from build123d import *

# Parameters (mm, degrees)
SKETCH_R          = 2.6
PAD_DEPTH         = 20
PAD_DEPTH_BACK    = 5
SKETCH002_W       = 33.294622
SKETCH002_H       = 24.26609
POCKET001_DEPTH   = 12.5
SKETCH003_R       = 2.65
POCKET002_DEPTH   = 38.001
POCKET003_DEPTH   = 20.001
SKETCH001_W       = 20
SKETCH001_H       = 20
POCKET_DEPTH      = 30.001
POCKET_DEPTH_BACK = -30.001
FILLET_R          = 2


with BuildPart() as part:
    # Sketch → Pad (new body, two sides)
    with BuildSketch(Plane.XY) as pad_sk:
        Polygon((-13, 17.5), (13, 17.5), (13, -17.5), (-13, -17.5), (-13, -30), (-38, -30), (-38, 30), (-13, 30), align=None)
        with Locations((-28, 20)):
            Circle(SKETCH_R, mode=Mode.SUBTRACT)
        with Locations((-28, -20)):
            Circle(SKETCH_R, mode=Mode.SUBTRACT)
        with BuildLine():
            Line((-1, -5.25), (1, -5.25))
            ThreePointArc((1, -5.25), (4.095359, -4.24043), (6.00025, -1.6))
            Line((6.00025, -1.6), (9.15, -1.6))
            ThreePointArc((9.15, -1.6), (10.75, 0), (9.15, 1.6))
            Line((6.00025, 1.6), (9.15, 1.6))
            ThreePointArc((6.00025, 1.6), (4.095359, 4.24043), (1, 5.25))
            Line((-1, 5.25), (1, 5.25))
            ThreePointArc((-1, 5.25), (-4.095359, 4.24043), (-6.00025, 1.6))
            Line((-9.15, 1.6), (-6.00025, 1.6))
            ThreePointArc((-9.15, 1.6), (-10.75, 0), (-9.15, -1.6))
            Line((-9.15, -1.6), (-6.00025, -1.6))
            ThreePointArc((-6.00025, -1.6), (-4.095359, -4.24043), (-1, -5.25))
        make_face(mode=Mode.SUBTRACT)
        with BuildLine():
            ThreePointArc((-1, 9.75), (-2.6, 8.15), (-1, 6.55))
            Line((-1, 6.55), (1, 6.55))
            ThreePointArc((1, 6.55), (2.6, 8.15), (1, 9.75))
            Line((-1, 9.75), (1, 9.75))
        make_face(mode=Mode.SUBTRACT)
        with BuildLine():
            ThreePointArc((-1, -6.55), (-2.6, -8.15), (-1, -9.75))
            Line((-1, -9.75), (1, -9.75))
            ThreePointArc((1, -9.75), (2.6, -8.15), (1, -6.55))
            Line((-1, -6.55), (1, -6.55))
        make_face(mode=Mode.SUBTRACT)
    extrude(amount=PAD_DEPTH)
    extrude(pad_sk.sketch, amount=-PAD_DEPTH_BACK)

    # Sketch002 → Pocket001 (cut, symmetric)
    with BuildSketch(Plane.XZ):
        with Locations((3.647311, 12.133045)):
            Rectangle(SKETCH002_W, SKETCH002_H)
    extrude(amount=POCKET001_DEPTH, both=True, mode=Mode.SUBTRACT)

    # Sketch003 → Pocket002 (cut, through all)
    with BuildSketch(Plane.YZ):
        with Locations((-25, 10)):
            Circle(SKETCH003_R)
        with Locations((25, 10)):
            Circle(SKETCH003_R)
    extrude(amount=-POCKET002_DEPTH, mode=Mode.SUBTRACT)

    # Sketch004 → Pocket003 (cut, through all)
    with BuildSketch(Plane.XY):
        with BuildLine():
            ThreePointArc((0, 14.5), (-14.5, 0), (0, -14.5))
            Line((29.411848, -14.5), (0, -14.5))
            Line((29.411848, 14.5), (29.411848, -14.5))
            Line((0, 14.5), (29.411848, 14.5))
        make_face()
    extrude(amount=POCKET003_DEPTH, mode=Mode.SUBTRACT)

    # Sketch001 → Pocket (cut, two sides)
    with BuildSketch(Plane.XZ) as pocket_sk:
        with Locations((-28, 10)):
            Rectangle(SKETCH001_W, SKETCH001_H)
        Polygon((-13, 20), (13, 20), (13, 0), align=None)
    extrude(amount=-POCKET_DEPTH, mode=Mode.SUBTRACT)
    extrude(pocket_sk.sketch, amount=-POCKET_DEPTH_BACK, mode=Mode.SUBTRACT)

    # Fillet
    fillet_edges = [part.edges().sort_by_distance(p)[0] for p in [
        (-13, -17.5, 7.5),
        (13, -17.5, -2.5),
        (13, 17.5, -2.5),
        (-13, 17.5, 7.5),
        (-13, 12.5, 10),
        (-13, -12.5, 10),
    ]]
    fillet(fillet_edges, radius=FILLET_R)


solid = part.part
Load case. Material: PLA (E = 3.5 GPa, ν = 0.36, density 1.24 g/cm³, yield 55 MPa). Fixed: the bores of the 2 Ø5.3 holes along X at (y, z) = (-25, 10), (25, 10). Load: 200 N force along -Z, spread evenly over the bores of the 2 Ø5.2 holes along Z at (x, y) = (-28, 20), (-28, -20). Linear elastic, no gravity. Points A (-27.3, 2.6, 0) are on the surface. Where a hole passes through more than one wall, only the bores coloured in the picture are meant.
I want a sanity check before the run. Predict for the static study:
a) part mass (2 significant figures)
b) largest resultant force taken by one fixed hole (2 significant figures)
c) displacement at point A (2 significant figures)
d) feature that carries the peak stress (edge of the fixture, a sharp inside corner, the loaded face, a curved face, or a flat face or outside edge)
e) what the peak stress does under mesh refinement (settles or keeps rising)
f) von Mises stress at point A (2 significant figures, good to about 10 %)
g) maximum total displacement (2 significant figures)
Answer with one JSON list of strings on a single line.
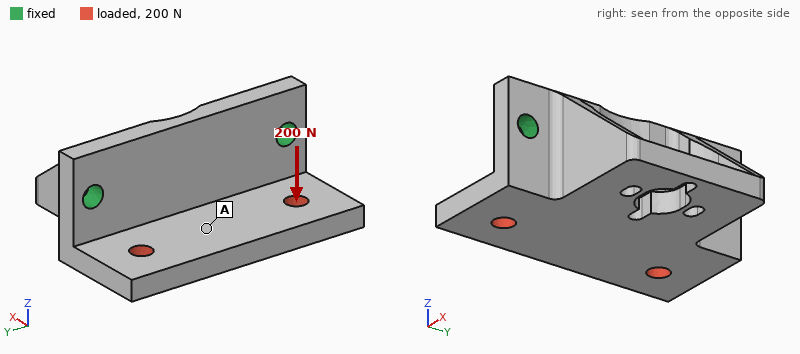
["23 g", "110 N", "0.17 mm", "edge of the fixture", "keeps rising", "2.5 MPa", "0.39 mm"]
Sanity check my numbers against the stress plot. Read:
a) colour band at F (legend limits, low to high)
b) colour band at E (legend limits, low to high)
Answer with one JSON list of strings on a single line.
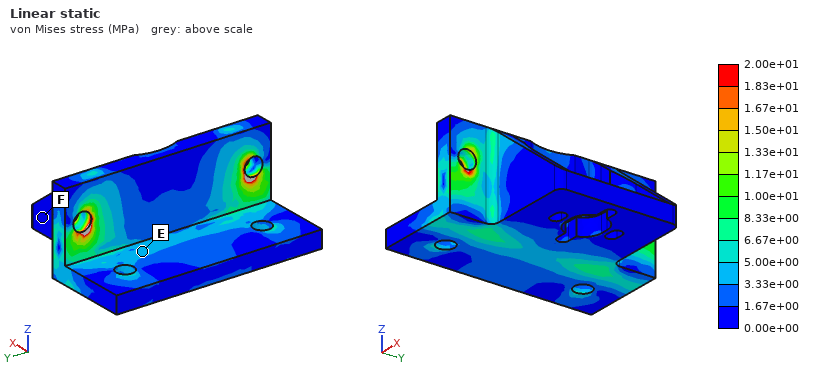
["0.00e+00 to 1.67e+00 MPa", "3.33e+00 to 5.00e+00 MPa"]
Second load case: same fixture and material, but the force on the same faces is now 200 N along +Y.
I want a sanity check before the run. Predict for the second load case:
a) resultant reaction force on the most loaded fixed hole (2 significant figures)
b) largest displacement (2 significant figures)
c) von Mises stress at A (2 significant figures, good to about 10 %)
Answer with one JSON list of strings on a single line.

["120 N", "63 µm", "1.5 MPa"]
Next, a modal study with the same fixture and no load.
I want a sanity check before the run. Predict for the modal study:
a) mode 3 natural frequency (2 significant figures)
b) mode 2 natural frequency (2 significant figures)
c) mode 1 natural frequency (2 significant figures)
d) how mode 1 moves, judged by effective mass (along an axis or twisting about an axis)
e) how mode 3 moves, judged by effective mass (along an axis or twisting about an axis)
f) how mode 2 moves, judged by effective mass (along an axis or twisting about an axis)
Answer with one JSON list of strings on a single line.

["2800 Hz", "2300 Hz", "1300 Hz", "along X", "along Z", "twisting about Z"]
